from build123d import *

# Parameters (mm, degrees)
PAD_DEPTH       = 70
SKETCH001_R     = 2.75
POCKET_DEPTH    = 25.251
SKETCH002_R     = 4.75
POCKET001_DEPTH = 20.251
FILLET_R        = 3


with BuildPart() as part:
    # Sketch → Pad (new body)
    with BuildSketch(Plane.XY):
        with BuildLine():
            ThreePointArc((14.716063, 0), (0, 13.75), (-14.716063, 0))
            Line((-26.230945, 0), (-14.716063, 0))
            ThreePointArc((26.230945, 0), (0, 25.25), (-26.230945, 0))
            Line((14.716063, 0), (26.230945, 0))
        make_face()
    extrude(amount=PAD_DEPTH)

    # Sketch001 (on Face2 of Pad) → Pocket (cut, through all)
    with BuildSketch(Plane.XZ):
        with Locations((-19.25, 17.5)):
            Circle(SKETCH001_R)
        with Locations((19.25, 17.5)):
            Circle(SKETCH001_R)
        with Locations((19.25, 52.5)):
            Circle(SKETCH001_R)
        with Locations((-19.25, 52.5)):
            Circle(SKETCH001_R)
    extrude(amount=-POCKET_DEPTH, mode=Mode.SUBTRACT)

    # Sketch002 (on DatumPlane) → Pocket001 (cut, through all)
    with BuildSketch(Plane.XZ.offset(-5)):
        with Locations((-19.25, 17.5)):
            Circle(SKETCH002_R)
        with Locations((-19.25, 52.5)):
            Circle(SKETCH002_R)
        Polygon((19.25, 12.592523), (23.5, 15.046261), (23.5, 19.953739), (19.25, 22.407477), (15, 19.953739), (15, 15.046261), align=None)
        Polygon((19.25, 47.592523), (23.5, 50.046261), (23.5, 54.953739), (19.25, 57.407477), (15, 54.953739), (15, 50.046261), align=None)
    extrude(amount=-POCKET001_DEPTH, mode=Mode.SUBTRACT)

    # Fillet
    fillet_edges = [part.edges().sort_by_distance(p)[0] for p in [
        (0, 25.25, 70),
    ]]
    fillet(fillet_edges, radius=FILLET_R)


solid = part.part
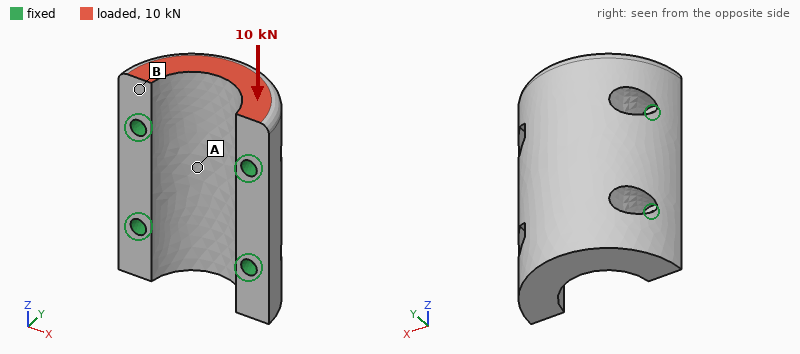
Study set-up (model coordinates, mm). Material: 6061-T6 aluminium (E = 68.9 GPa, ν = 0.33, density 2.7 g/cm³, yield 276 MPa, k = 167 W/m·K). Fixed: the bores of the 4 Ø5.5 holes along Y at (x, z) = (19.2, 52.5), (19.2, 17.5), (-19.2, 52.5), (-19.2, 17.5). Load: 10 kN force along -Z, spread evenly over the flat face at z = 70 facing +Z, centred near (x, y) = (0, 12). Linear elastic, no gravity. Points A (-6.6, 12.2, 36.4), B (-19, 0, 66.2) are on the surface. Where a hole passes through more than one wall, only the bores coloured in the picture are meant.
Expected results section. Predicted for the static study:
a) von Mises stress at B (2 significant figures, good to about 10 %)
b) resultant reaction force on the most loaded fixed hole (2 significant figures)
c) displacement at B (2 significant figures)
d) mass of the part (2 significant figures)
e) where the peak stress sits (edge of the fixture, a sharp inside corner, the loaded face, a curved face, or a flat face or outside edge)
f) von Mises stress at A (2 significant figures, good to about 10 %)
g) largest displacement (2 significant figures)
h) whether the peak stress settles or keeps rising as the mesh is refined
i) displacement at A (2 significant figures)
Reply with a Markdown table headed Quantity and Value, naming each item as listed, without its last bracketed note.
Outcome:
| Quantity | Value |
|---|---|
| von Mises stress at B | 24 MPa |
| resultant reaction force on the most loaded fixed hole | 3.6 kN |
| displacement at B | 9.4 µm |
| mass of the part | 130 g |
| where the peak stress sits | edge of the fixture |
| von Mises stress at A | 9.8 MPa |
| largest displacement | 20 µm |
| whether the peak stress settles or keeps rising as the mesh is refined | keeps rising |
| displacement at A | 7.7 µm |
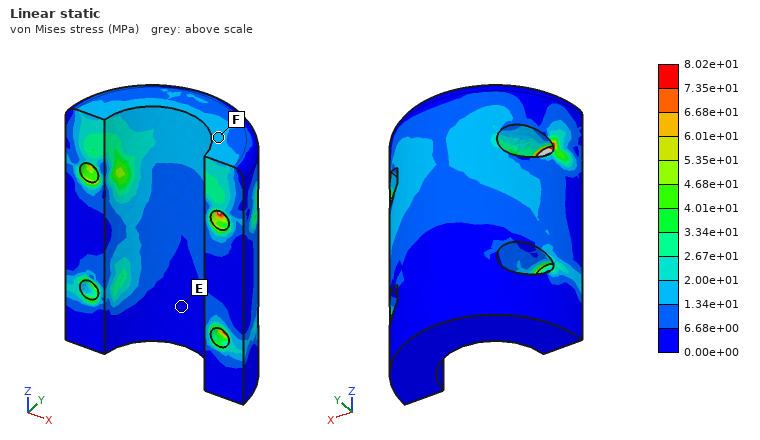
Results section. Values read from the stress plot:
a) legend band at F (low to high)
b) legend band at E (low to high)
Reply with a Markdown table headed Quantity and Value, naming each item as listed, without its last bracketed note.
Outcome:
| Quantity | Value |
|---|---|
| legend band at F | 1.34e+01 to 2.00e+01 MPa |
| legend band at E | 0.00e+00 to 6.68e+00 MPa |
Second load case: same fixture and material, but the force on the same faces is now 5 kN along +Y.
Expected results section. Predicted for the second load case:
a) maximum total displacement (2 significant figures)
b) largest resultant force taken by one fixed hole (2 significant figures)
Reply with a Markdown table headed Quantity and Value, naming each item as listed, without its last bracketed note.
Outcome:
| Quantity | Value |
|---|---|
| maximum total displacement | 36 µm |
| largest resultant force taken by one fixed hole | 3.9 kN |
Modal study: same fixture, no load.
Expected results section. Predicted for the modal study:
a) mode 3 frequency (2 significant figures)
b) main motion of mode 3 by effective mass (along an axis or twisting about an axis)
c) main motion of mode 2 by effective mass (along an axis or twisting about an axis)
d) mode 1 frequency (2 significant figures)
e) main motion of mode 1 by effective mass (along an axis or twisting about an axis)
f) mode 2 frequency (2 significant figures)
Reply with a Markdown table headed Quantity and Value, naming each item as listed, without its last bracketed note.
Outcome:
| Quantity | Value |
|---|---|
| mode 3 frequency | 15 kHz |
| main motion of mode 3 by effective mass | twisting about Y |
| main motion of mode 2 by effective mass | along X |
| mode 1 frequency | 11 kHz |
| main motion of mode 1 by effective mass | along Z |
| mode 2 frequency | 13 kHz |
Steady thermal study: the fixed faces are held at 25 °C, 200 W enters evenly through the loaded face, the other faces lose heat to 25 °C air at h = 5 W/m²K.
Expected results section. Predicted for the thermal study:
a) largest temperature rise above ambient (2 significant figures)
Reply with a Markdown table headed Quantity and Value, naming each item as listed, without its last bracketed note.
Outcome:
| Quantity | Value |
|---|---|
| largest temperature rise above ambient | 61 K |
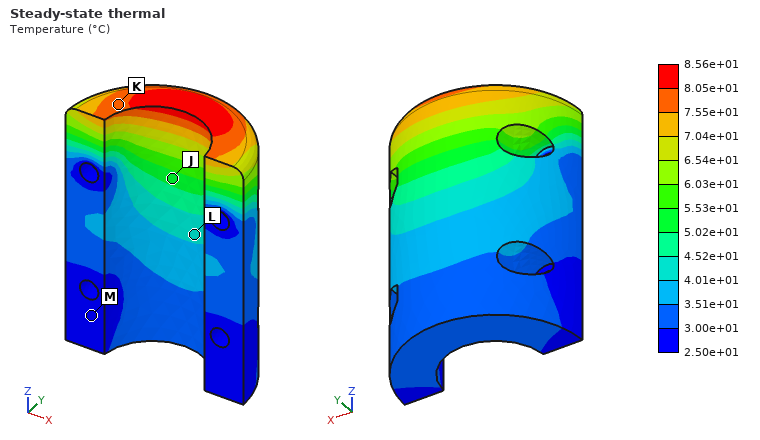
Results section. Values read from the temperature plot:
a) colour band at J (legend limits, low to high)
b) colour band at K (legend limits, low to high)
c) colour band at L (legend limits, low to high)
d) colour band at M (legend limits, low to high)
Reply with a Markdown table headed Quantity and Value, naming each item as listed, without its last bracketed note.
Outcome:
| Quantity | Value |
|---|---|
| colour band at J | 5.02e+01 to 5.53e+01 °C |
| colour band at K | 7.55e+01 to 8.05e+01 °C |
| colour band at L | 4.01e+01 to 4.52e+01 °C |
| colour band at M | 2.50e+01 to 3.00e+01 °C |
